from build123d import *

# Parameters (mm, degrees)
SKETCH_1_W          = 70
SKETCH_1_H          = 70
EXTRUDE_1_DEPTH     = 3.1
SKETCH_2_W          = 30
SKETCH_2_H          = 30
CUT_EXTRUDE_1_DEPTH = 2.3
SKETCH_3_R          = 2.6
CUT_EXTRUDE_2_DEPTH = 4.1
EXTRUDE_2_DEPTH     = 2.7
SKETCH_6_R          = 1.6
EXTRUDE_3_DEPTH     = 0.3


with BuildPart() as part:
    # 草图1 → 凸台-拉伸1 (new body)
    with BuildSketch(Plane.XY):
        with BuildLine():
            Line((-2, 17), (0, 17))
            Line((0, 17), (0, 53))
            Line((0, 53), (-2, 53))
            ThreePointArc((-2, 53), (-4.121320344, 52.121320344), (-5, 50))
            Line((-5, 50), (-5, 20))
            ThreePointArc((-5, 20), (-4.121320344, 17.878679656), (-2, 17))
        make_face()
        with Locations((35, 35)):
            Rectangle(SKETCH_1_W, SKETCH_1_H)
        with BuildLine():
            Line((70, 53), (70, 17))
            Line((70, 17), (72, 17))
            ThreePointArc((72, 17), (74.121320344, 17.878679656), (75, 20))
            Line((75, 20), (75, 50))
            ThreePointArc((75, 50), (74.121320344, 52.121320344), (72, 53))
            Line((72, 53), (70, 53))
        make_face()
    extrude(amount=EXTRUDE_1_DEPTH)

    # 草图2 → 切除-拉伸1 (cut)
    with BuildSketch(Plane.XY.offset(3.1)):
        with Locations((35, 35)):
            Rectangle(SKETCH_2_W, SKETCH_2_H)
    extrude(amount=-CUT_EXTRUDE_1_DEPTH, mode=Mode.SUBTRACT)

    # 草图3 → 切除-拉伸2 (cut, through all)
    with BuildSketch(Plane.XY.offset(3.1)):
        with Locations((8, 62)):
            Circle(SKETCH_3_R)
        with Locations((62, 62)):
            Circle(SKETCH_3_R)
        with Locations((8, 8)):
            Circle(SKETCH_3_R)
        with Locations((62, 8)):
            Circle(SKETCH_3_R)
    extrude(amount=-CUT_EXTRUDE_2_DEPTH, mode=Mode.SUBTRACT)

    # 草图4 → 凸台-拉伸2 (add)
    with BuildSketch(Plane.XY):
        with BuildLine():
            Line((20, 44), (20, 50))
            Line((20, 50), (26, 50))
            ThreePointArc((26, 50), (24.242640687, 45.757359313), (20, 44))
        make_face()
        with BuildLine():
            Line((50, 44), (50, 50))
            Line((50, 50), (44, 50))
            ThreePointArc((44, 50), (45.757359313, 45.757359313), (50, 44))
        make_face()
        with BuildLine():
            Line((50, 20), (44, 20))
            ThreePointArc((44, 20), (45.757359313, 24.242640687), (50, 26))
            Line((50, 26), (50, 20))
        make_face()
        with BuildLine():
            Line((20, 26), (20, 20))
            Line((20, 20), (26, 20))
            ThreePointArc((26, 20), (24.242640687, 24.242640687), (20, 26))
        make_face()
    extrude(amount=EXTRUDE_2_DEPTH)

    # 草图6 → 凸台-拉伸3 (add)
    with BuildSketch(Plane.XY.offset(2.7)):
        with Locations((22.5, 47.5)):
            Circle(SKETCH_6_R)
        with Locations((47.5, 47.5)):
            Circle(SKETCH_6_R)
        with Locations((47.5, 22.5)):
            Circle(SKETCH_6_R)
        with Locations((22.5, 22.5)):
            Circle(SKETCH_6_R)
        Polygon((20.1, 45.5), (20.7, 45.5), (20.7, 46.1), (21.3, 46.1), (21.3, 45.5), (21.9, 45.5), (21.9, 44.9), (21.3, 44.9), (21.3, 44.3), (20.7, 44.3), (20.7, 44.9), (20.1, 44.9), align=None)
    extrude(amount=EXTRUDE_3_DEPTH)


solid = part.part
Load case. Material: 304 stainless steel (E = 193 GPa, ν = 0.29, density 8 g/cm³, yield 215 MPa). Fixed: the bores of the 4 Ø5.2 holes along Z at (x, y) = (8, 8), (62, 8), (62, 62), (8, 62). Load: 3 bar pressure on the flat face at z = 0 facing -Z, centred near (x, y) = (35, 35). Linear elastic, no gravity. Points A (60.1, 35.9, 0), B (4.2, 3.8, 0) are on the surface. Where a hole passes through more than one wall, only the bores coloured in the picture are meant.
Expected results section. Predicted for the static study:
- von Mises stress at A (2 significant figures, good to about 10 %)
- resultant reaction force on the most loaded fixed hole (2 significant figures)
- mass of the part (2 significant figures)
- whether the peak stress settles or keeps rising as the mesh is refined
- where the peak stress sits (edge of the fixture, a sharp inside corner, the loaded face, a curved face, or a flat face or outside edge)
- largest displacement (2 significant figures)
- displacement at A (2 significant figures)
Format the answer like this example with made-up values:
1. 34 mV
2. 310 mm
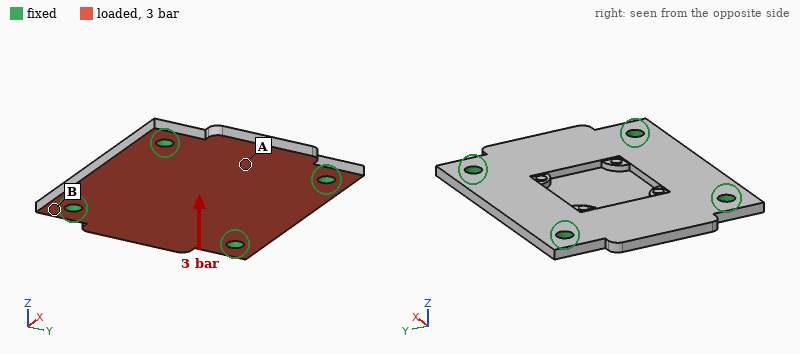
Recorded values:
1. 30 MPa
2. 420 N
3. 110 g
4. keeps rising
5. edge of the fixture
6. 71 µm
7. 20 µm
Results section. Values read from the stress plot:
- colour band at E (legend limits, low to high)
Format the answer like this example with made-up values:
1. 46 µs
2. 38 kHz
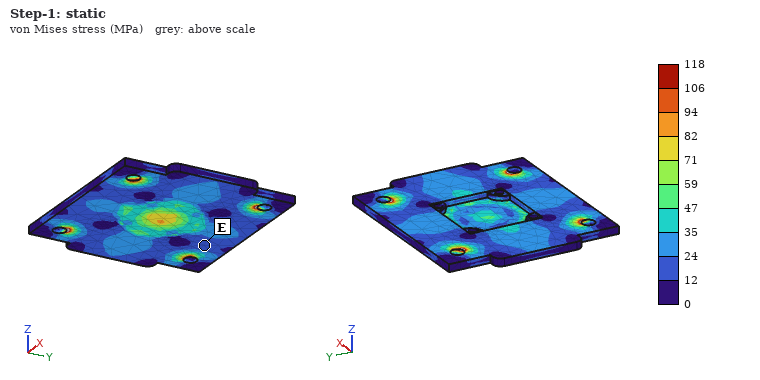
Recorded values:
1. 12 to 24 MPa
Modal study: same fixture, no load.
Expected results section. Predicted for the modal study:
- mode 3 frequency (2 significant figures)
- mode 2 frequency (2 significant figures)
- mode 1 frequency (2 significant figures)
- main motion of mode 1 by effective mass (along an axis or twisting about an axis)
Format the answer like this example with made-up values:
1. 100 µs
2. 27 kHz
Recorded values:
1. 5400 Hz
2. 5300 Hz
3. 4400 Hz
4. along Z
